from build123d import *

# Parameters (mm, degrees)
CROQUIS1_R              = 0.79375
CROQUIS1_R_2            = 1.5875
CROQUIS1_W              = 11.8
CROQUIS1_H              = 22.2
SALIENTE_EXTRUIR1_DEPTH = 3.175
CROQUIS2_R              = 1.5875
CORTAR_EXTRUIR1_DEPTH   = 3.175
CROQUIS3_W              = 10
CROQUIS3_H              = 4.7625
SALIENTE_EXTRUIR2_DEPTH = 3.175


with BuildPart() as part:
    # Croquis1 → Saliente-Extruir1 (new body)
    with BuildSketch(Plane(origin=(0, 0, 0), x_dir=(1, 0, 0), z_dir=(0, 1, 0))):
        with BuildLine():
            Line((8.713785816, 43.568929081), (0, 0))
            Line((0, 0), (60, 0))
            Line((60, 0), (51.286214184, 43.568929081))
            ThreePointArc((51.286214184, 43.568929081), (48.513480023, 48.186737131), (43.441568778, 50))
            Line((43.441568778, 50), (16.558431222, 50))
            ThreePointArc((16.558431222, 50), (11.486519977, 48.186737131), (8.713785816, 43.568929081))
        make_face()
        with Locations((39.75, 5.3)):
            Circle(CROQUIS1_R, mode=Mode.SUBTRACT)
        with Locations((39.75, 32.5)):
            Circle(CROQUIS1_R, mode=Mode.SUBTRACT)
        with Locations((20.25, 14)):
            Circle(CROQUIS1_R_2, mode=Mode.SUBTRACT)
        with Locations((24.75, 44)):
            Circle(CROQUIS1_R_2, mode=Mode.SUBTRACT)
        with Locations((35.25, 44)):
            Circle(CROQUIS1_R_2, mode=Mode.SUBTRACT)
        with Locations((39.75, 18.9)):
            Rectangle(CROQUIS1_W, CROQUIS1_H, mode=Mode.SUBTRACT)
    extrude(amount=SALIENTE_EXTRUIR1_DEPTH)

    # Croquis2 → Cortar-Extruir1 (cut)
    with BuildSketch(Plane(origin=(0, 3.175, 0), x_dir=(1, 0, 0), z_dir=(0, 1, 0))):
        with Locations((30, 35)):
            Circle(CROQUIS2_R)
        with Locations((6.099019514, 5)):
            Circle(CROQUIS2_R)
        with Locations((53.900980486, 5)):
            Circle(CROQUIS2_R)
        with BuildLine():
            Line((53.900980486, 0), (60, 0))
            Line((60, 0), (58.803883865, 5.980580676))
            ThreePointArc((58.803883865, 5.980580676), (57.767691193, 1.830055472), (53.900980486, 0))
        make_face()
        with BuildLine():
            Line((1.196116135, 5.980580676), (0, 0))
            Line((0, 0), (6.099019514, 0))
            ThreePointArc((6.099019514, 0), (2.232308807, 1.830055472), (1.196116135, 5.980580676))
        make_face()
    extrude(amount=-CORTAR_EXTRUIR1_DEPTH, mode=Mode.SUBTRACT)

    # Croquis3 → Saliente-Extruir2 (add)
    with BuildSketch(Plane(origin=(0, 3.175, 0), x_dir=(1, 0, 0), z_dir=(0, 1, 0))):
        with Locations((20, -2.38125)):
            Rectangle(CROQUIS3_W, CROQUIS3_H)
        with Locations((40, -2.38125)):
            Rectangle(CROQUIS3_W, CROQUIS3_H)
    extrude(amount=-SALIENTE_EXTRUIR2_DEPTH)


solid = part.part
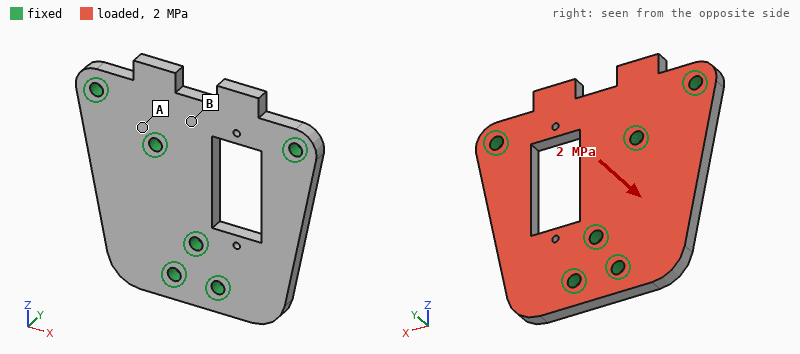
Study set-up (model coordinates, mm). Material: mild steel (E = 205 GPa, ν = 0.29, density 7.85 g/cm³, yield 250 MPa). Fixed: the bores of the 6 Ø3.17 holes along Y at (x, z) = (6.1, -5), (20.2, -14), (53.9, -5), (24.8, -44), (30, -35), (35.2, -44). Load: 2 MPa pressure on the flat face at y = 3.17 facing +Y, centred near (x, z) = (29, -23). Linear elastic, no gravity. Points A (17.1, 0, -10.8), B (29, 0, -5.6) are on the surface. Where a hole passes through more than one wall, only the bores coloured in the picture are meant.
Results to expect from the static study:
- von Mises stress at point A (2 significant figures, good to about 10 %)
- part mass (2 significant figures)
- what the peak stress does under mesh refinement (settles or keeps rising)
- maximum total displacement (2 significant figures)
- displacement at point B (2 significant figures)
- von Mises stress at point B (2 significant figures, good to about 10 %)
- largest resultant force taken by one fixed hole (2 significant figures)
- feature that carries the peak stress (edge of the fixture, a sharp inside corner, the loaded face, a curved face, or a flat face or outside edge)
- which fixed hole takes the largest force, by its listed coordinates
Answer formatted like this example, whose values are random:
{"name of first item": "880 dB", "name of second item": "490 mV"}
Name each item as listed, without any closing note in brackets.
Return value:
{"von Mises stress at point A": "89 MPa", "part mass": "56 g", "what the peak stress does under mesh refinement": "keeps rising", "maximum total displacement": "46 µm", "displacement at point B": "17 µm", "von Mises stress at point B": "36 MPa", "largest resultant force taken by one fixed hole": "1.3 kN", "feature that carries the peak stress": "edge of the fixture", "which fixed hole takes the largest force, by its listed coordinates": "(20.2, -14)"}
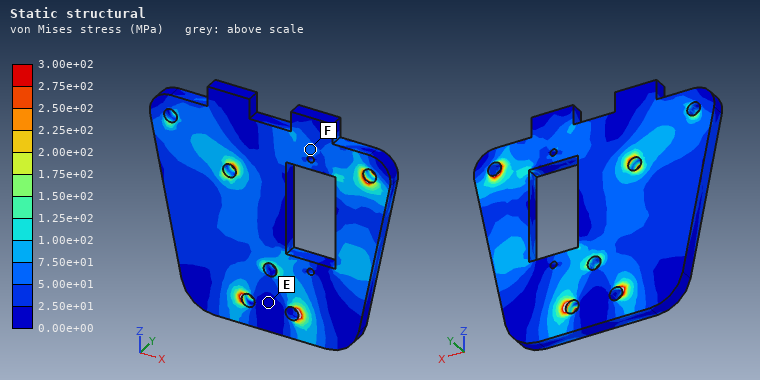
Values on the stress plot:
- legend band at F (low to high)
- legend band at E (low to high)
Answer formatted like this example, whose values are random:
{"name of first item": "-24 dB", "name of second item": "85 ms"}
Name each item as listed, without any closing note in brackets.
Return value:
{"legend band at F": "5.00e+01 to 7.50e+01 MPa", "legend band at E": "0.00e+00 to 2.50e+01 MPa"}
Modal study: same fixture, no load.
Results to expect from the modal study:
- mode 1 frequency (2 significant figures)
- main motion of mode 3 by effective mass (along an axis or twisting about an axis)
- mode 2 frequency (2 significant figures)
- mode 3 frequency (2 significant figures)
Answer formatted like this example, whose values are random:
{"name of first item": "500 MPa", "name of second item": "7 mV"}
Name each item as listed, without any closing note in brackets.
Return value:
{"mode 1 frequency": "8300 Hz", "main motion of mode 3 by effective mass": "along Y", "mode 2 frequency": "9400 Hz", "mode 3 frequency": "10 kHz"}
